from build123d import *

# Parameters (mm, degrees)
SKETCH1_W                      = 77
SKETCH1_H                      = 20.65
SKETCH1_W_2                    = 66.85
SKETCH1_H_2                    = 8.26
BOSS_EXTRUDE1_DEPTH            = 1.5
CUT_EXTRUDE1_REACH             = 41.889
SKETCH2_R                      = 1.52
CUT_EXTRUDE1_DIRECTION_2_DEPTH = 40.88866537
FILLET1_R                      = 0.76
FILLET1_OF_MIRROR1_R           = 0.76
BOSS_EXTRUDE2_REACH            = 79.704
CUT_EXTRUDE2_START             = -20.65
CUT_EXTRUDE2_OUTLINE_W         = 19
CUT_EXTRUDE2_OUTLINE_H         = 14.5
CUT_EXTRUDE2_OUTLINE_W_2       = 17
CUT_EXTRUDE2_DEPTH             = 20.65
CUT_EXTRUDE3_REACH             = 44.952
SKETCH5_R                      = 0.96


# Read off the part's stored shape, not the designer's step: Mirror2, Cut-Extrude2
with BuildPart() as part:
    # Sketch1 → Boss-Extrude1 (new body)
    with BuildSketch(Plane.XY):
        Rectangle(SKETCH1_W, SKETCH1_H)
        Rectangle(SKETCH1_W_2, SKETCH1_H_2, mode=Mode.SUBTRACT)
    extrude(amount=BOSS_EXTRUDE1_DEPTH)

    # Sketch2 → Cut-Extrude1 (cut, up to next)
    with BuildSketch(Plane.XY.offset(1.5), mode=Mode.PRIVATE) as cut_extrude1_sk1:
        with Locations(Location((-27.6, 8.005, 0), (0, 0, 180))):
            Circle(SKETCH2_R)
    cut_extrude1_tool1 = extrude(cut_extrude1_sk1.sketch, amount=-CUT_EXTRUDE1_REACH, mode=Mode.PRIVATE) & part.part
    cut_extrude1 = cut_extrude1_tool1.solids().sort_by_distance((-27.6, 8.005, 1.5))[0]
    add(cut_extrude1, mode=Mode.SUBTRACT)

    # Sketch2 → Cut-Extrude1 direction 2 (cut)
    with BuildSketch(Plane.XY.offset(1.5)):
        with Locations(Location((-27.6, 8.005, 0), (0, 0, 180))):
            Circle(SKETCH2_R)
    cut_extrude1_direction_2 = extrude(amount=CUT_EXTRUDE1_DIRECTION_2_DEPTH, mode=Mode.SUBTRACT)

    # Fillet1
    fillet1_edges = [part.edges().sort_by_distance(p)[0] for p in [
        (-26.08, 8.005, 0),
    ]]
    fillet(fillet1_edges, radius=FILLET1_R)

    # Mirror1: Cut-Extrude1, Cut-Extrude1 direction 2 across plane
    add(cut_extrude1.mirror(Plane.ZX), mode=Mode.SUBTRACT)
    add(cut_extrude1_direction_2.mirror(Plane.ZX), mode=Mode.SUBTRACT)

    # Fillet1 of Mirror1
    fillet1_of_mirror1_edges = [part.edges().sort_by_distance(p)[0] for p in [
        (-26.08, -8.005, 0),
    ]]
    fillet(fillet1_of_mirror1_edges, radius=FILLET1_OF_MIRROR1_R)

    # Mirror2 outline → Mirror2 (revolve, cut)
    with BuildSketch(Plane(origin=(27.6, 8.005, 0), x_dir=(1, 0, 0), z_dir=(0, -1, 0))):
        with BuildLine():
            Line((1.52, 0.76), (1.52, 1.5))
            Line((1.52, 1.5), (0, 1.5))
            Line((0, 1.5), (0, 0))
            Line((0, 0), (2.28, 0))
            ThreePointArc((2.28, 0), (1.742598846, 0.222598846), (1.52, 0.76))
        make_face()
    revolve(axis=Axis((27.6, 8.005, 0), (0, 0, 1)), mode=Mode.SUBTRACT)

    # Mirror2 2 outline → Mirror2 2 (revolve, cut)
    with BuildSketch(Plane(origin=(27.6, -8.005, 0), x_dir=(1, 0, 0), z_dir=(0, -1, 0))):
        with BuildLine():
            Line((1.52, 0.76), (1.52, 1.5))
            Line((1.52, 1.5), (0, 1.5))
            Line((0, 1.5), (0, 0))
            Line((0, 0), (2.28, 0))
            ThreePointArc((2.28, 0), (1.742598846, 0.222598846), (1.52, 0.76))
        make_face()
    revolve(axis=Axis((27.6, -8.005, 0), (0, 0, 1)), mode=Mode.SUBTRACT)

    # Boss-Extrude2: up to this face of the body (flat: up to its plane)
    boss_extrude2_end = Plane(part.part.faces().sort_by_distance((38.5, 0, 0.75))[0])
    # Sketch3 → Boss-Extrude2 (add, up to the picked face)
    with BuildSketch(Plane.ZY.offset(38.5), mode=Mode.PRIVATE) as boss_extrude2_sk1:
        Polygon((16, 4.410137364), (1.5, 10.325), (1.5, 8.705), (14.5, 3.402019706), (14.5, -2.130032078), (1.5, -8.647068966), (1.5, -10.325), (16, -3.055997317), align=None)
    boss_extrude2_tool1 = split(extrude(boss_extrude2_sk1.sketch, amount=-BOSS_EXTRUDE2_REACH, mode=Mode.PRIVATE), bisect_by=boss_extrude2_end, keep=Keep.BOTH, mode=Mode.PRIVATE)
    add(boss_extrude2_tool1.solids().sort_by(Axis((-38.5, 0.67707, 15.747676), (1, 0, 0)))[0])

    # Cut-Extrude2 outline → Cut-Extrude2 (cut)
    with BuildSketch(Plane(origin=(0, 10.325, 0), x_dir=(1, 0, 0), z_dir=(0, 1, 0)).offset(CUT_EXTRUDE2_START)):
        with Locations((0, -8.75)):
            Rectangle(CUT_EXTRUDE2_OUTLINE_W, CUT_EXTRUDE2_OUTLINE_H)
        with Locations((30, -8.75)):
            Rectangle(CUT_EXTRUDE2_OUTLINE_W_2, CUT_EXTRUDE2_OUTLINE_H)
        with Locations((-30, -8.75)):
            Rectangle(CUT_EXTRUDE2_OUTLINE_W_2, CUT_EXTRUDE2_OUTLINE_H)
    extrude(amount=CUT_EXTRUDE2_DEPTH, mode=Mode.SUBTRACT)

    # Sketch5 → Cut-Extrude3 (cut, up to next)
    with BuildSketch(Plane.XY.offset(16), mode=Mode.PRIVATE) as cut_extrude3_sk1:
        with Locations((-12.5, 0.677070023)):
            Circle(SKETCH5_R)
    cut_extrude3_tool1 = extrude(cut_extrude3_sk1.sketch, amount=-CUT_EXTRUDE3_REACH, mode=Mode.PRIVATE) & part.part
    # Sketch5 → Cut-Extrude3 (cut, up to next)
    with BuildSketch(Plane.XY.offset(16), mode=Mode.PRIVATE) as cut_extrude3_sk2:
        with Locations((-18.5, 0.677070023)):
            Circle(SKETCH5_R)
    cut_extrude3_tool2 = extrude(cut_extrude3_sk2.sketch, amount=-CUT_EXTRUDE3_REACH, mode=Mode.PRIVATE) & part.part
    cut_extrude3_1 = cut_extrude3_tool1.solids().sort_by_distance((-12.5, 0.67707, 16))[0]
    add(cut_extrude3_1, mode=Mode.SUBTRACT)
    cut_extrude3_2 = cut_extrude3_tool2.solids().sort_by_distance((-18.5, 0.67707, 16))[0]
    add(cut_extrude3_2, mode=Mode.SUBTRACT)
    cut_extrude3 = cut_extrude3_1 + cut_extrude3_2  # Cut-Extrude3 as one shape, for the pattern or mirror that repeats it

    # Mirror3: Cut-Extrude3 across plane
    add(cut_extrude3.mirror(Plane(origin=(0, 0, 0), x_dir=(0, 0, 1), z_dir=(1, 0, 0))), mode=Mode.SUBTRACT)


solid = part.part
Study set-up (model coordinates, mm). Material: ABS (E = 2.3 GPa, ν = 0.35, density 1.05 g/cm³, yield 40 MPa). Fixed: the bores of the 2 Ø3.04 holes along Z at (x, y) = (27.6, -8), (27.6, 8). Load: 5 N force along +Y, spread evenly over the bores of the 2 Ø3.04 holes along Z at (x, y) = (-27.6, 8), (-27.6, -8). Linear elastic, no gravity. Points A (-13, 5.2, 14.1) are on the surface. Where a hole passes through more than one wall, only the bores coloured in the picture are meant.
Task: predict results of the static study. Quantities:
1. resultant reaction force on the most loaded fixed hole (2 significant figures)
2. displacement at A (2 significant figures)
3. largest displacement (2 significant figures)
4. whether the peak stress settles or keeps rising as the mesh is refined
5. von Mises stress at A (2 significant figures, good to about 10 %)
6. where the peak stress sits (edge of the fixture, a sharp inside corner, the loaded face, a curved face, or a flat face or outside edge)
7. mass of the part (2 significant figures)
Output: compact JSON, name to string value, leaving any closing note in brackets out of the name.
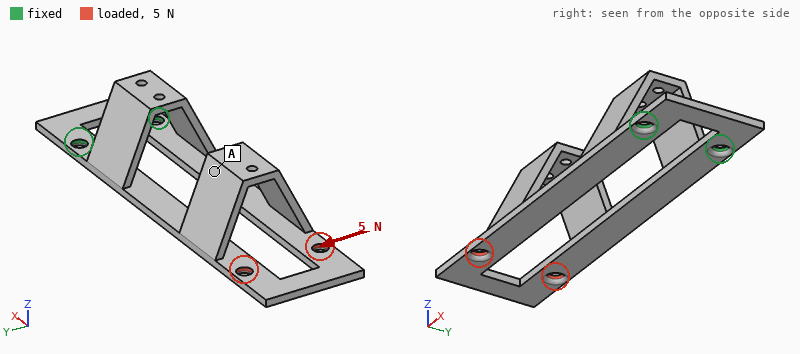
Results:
{"resultant reaction force on the most loaded fixed hole": "10 N", "displacement at A": "0.43 mm", "largest displacement": "0.85 mm", "whether the peak stress settles or keeps rising as the mesh is refined": "keeps rising", "von Mises stress at A": "1.2 MPa", "where the peak stress sits": "edge of the fixture", "mass of the part": "3.0 g"}
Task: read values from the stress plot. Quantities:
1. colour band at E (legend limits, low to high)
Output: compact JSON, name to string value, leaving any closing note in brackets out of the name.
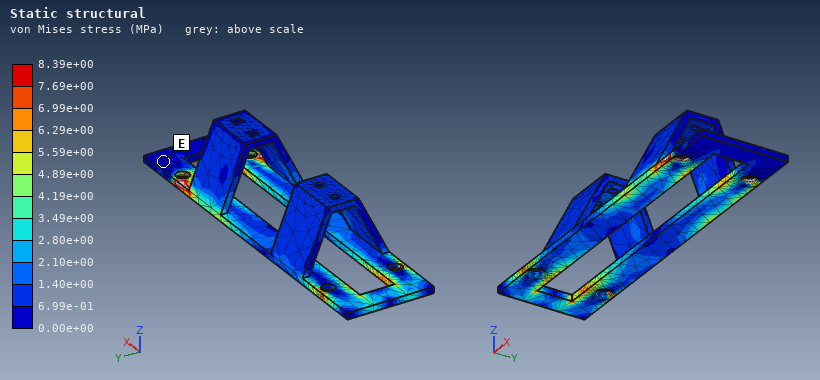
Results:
{"colour band at E": "0.00e+00 to 6.99e-01 MPa"}
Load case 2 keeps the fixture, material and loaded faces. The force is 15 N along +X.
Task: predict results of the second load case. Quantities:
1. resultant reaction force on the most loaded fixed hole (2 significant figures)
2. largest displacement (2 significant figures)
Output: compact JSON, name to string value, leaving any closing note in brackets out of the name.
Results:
{"resultant reaction force on the most loaded fixed hole": "7.5 N", "largest displacement": "0.93 mm"}
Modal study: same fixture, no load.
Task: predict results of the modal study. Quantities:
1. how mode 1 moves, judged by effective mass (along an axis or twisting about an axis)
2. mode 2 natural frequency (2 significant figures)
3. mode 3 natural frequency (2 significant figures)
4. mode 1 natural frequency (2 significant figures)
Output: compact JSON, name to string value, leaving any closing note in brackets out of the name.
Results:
{"how mode 1 moves, judged by effective mass": "along Z", "mode 2 natural frequency": "370 Hz", "mode 3 natural frequency": "380 Hz", "mode 1 natural frequency": "73 Hz"}
